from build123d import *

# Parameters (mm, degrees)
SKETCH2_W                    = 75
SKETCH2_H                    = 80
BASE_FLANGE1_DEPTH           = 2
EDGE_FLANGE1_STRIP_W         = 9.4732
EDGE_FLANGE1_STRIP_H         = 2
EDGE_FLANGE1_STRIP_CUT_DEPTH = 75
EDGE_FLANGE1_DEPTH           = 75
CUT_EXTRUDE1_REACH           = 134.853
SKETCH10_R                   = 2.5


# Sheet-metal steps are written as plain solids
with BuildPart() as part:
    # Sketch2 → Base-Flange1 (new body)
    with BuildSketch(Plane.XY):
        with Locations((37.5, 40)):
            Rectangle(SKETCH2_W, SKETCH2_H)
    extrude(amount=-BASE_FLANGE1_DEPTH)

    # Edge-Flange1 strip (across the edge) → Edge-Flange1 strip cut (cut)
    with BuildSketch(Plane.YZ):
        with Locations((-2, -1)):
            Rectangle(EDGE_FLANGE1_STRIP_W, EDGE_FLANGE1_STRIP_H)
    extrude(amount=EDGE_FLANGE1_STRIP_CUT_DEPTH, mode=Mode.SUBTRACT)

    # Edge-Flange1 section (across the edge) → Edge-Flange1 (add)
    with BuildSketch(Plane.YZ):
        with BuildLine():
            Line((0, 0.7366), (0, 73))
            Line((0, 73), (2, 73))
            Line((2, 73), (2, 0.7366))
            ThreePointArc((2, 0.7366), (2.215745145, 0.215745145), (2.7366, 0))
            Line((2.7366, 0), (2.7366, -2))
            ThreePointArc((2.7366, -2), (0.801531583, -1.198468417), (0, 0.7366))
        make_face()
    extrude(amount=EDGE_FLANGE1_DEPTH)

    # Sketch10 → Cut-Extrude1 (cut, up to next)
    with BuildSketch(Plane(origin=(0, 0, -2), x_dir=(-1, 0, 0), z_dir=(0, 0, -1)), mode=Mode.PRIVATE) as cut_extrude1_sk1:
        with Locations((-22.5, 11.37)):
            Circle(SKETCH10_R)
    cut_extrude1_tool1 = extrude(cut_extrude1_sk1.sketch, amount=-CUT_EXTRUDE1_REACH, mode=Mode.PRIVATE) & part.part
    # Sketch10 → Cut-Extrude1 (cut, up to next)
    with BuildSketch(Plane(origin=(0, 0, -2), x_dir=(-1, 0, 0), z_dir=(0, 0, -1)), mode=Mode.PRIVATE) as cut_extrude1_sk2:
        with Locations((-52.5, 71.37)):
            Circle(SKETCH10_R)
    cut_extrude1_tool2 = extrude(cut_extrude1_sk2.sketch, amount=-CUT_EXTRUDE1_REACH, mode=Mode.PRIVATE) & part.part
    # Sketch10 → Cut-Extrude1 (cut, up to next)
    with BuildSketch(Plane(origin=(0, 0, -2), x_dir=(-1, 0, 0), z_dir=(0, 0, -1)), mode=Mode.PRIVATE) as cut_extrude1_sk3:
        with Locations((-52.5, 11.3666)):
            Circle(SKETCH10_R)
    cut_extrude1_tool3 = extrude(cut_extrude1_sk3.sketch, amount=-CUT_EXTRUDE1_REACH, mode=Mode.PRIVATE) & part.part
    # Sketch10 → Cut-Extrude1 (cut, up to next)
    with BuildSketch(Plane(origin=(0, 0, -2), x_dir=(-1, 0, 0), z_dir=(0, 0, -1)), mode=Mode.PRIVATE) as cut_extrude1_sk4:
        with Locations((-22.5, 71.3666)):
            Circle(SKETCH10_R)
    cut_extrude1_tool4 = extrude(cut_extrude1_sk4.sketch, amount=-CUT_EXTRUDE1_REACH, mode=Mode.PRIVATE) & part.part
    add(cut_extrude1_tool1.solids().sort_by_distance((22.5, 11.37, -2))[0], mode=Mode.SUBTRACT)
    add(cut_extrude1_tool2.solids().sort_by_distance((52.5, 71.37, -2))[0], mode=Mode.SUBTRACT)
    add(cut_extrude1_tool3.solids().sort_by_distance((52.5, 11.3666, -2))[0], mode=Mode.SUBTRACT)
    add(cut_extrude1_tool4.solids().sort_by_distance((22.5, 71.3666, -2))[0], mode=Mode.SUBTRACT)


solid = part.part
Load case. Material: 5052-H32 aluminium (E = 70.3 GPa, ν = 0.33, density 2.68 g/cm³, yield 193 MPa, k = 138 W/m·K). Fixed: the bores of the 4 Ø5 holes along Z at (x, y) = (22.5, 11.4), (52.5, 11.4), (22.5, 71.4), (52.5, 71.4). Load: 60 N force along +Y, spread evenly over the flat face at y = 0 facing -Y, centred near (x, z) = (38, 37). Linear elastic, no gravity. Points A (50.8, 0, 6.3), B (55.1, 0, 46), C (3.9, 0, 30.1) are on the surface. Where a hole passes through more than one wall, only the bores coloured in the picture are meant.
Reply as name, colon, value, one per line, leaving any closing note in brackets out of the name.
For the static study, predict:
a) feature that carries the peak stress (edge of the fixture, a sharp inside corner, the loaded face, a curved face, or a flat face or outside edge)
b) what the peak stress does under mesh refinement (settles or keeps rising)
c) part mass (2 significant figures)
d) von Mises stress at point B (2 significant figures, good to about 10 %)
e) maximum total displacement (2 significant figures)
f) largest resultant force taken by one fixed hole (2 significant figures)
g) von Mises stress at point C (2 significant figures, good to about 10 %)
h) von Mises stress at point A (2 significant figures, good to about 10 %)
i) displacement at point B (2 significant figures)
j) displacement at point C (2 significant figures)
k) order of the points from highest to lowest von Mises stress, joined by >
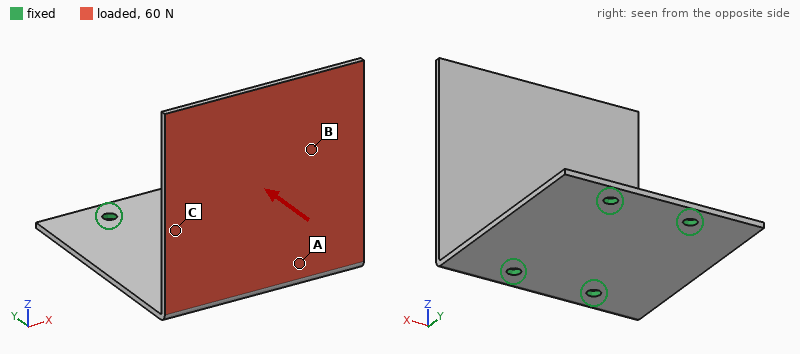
feature that carries the peak stress: edge of the fixture
what the peak stress does under mesh refinement: keeps rising
part mass: 61 g
von Mises stress at point B: 5.9 MPa
maximum total displacement: 1.3 mm
largest resultant force taken by one fixed hole: 26 N
von Mises stress at point C: 15 MPa
von Mises stress at point A: 34 MPa
displacement at point B: 0.71 mm
displacement at point C: 0.40 mm
order of the points from highest to lowest von Mises stress, joined by >: A > C > B
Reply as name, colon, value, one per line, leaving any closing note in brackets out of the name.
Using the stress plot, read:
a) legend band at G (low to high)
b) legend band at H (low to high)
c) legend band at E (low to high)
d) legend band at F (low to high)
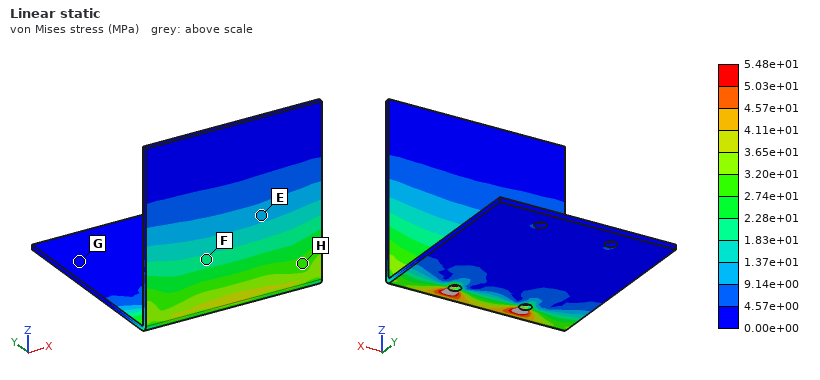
legend band at G: 0.00e+00 to 4.57e+00 MPa
legend band at H: 2.74e+01 to 3.20e+01 MPa
legend band at E: 9.14e+00 to 1.37e+01 MPa
legend band at F: 1.83e+01 to 2.28e+01 MPa
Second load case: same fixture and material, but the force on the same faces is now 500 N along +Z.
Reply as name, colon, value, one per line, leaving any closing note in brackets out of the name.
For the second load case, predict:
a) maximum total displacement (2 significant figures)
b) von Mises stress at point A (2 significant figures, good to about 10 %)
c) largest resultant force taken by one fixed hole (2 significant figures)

maximum total displacement: 0.92 mm
von Mises stress at point A: 14 MPa
largest resultant force taken by one fixed hole: 260 N
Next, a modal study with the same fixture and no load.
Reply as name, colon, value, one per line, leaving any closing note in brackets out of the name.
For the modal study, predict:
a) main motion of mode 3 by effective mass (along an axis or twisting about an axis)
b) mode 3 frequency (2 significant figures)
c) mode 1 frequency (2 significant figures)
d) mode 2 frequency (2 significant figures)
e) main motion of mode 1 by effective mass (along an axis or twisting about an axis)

main motion of mode 3 by effective mass: along X
mode 3 frequency: 1200 Hz
mode 1 frequency: 250 Hz
mode 2 frequency: 660 Hz
main motion of mode 1 by effective mass: along Y
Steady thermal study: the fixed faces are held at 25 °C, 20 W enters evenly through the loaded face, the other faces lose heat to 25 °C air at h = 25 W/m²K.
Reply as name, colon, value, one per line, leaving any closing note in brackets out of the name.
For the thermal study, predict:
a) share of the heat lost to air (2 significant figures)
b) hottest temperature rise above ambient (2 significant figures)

share of the heat lost to air: 26 %
hottest temperature rise above ambient: 38 K
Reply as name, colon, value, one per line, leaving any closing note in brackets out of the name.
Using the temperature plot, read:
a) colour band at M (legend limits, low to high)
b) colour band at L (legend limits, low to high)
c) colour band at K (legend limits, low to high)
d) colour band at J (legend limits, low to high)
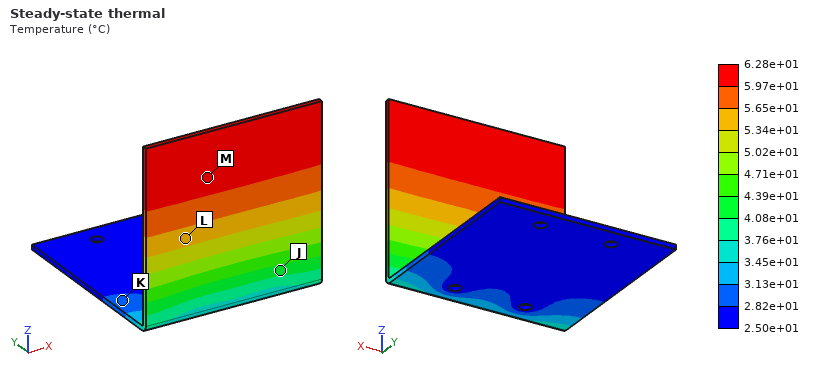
colour band at M: 5.97e+01 to 6.28e+01 °C
colour band at L: 5.34e+01 to 5.65e+01 °C
colour band at K: 2.82e+01 to 3.13e+01 °C
colour band at J: 4.08e+01 to 4.39e+01 °C
